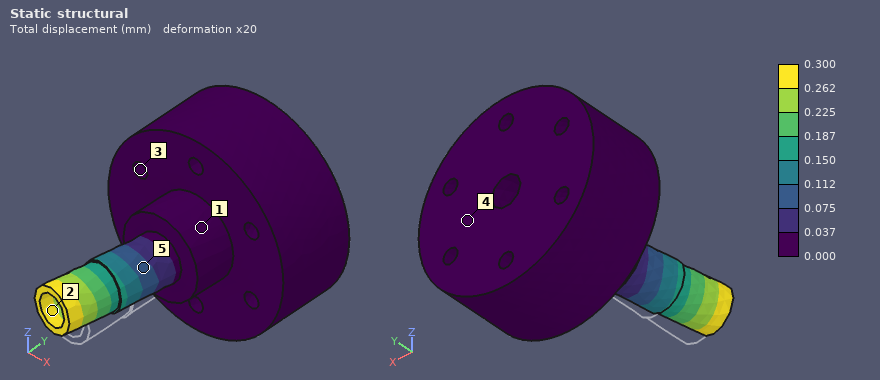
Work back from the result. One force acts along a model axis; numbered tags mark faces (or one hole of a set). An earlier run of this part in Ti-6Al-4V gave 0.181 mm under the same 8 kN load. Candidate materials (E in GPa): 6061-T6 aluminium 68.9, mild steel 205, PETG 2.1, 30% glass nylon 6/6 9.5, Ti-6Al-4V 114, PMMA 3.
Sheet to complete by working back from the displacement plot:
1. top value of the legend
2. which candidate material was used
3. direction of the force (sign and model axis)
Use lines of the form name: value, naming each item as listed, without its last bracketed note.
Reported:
top value of the legend: 0.300 mm
which candidate material was used: 6061-T6 aluminium
direction of the force: -X
